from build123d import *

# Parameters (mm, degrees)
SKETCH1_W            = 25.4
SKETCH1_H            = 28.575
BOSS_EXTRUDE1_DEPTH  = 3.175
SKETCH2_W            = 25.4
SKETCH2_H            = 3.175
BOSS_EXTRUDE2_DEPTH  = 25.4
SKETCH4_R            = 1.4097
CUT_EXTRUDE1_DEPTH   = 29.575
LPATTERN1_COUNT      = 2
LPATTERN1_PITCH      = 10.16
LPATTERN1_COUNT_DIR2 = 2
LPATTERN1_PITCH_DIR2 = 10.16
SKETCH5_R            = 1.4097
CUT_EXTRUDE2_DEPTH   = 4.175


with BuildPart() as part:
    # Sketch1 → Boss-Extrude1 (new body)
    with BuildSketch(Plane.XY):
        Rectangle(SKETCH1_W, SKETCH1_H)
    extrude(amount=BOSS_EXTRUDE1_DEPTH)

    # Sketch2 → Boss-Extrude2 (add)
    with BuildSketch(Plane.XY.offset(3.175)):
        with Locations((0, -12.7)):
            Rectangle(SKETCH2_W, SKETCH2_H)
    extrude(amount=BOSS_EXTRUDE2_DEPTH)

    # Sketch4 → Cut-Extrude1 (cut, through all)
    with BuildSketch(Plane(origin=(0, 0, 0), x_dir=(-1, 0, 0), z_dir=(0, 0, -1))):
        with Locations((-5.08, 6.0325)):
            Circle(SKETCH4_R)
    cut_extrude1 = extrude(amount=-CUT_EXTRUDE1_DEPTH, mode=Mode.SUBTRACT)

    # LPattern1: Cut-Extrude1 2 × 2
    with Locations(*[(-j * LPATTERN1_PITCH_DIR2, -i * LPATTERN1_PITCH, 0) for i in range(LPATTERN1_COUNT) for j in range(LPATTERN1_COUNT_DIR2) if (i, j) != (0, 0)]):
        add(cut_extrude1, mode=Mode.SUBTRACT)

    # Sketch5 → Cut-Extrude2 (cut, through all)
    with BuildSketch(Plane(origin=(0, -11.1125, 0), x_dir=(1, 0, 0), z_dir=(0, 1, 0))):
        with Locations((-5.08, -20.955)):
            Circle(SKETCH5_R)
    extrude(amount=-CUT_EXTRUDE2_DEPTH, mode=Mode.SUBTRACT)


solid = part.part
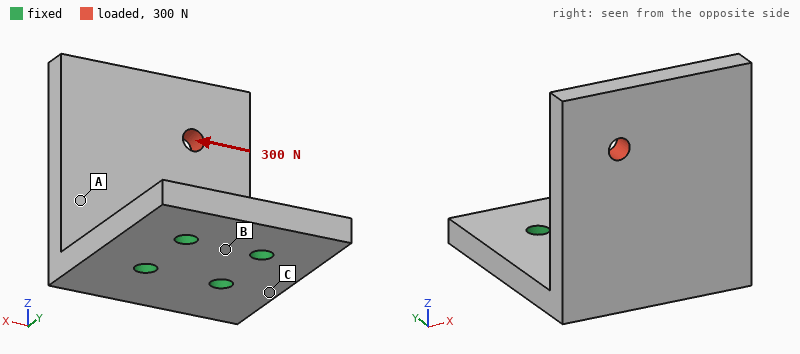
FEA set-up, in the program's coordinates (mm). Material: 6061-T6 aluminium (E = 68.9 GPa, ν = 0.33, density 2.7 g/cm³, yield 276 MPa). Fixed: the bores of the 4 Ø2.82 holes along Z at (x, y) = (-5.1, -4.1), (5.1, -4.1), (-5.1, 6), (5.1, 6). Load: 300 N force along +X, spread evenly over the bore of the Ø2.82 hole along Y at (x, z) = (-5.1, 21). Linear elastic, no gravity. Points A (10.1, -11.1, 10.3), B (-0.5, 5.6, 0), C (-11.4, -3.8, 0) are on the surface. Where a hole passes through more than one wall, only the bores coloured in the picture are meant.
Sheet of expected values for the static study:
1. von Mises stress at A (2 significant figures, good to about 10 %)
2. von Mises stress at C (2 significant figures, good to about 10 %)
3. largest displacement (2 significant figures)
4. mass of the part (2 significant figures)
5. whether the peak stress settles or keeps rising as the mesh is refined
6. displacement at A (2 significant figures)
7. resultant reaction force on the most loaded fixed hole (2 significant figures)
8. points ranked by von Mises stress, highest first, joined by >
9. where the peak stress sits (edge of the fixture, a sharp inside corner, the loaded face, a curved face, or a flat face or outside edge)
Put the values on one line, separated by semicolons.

23 MPa; 46 MPa; 92 µm; 11 g; keeps rising; 41 µm; 480 N; C > A > B; edge of the fixture
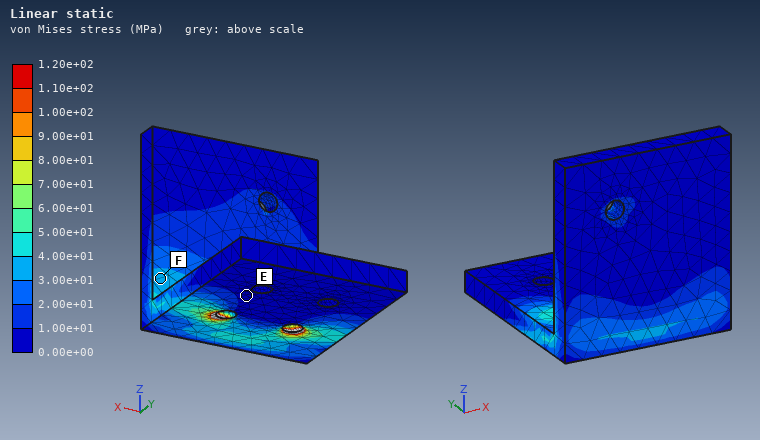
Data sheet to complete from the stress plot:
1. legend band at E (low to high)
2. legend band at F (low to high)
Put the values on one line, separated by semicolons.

0.00e+00 to 1.00e+01 MPa; 3.00e+01 to 4.00e+01 MPa
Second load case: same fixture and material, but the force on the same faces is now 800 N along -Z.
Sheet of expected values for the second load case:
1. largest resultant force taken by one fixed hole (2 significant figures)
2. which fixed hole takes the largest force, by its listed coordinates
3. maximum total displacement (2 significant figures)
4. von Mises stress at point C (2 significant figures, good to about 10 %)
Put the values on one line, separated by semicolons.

780 N; (-5.1, -4.1); 0.20 mm; 85 MPa
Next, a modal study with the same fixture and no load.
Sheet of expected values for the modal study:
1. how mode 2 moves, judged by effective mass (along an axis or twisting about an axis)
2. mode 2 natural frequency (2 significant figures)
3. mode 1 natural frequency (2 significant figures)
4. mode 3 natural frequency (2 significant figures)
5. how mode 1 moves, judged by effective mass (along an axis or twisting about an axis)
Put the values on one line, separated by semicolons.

along X; 5200 Hz; 2500 Hz; 8400 Hz; along Y
